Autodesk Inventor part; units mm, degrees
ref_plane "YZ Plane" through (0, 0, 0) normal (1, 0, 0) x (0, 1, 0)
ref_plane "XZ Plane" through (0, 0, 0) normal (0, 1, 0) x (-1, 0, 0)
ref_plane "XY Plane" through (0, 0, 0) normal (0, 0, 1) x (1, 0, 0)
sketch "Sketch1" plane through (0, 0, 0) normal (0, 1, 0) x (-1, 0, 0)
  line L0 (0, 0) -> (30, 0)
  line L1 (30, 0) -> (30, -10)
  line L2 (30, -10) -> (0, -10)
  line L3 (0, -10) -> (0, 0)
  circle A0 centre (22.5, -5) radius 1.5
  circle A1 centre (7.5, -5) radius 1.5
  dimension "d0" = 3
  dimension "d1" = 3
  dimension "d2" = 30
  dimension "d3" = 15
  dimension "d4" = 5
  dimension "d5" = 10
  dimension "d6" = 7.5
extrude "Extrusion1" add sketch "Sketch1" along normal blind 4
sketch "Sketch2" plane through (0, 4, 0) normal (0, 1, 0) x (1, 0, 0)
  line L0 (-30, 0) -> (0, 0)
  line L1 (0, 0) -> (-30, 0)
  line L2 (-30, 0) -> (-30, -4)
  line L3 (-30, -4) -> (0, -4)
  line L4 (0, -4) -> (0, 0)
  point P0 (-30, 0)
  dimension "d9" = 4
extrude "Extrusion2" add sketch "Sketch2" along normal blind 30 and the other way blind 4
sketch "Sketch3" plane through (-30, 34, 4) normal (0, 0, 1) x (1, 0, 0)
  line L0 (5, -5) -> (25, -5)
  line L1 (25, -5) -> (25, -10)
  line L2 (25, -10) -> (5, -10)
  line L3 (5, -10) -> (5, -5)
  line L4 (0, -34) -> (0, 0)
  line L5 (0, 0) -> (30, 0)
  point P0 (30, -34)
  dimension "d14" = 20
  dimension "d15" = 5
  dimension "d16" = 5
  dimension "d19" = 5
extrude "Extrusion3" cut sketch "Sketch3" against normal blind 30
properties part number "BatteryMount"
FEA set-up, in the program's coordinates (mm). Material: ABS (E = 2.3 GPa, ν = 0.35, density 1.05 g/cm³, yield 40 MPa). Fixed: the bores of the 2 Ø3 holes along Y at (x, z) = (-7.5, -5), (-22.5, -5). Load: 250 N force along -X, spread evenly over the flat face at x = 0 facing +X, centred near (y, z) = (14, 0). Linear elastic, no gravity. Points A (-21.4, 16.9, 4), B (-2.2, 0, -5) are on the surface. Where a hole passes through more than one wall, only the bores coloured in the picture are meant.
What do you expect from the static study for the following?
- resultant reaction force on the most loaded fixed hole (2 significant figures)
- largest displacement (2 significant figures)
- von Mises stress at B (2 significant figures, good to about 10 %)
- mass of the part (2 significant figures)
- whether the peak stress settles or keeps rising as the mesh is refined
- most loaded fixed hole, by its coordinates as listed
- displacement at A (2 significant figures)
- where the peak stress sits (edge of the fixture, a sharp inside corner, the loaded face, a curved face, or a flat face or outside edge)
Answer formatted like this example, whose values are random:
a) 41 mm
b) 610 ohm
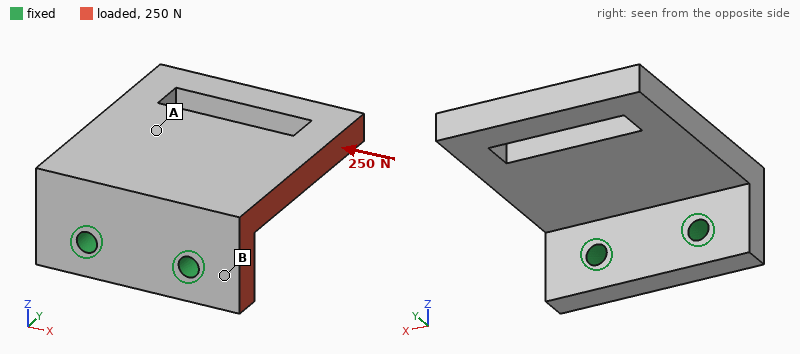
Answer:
a) 230 N
b) 0.51 mm
c) 8.9 MPa
d) 5.1 g
e) keeps rising
f) (-7.5, -5)
g) 0.19 mm
h) edge of the fixture
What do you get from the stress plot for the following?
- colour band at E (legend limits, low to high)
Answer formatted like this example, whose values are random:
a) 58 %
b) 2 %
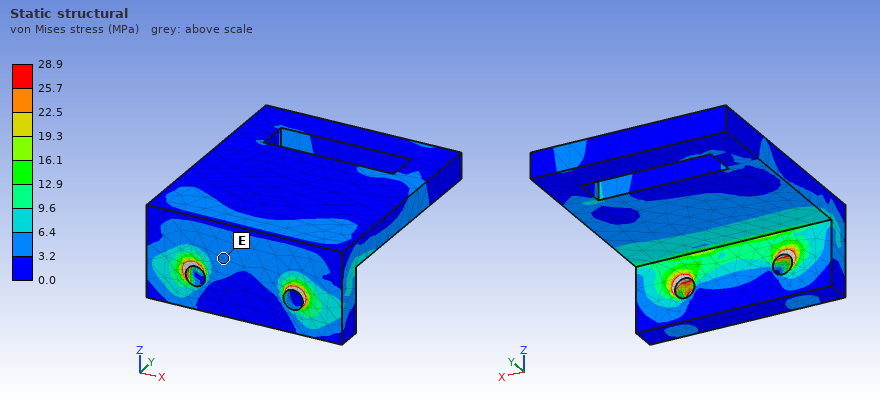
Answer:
a) 3.2 to 6.4 MPa
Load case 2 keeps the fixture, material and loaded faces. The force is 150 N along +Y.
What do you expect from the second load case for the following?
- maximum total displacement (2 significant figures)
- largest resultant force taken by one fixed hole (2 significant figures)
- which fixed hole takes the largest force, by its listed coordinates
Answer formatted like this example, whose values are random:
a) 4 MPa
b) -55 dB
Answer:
a) 0.48 mm
b) 190 N
c) (-7.5, -5)
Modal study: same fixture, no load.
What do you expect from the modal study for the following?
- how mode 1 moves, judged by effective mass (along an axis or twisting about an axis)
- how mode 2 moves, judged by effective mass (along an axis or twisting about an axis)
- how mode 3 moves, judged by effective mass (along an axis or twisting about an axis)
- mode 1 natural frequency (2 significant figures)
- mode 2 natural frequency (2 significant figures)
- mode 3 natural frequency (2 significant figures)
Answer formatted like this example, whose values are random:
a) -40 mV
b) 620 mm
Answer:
a) along Z
b) along X
c) along X
d) 780 Hz
e) 1800 Hz
f) 2300 Hz
